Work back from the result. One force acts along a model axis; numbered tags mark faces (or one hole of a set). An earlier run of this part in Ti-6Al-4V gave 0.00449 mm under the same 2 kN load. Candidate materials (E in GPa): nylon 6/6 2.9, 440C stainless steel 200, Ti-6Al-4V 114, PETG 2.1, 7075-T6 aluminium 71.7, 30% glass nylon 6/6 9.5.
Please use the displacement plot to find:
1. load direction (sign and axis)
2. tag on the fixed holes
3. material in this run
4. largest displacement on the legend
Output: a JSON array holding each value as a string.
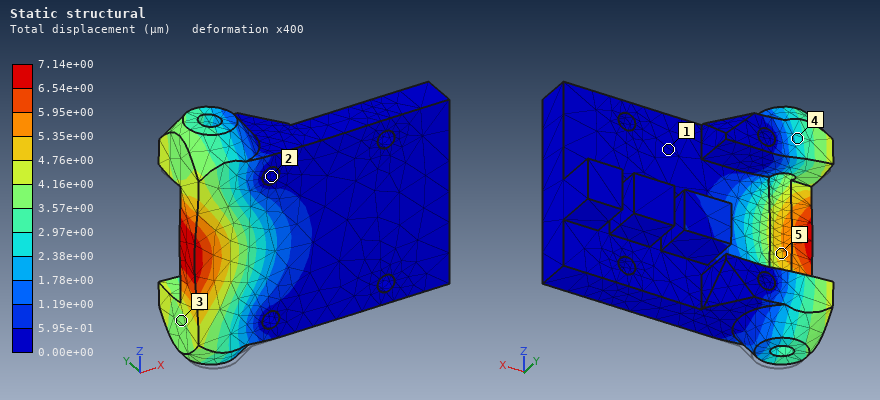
["+Y", "2", "7075-T6 aluminium", "7.14e+00 µm"]
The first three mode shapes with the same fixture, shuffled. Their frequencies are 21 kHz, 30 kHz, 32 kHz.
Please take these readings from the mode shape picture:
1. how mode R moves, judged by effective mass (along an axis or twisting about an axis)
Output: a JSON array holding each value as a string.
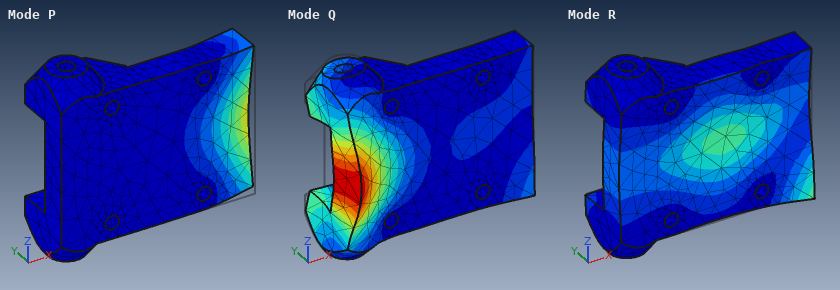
["along Y"]
